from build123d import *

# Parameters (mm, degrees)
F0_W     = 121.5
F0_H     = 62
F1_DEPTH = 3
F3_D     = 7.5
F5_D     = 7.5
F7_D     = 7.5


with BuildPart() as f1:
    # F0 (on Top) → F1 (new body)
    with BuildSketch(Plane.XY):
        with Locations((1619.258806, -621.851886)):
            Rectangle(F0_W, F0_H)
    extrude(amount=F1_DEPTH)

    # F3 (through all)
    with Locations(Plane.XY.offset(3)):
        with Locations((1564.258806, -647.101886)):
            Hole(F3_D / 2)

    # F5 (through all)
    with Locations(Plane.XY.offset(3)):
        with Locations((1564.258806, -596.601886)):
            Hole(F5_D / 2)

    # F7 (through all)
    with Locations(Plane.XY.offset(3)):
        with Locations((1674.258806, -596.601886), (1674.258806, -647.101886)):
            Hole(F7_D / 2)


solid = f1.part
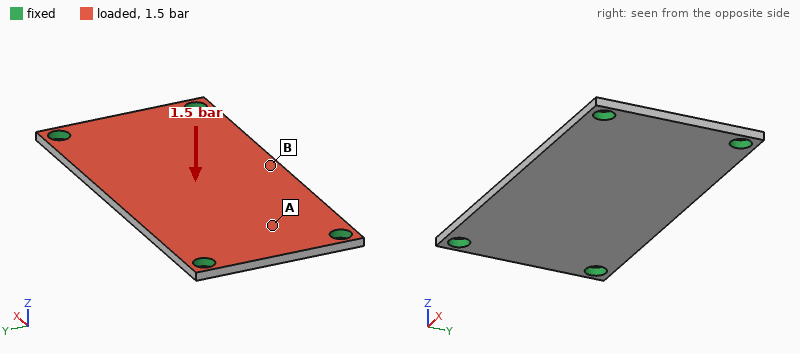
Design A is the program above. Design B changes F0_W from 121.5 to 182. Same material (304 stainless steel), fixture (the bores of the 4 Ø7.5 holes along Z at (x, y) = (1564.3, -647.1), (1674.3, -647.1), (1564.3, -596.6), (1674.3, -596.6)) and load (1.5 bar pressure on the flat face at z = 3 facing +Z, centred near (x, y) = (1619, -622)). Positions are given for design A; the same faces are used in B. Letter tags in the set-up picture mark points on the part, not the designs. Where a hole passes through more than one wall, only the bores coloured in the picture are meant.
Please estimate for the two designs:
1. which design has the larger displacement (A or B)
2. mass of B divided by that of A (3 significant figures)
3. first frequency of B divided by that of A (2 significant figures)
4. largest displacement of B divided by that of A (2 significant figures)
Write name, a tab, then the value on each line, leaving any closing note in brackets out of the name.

which design has the larger displacement	A
mass of B divided by that of A	1.51
first frequency of B divided by that of A	1.0
largest displacement of B divided by that of A	0.91
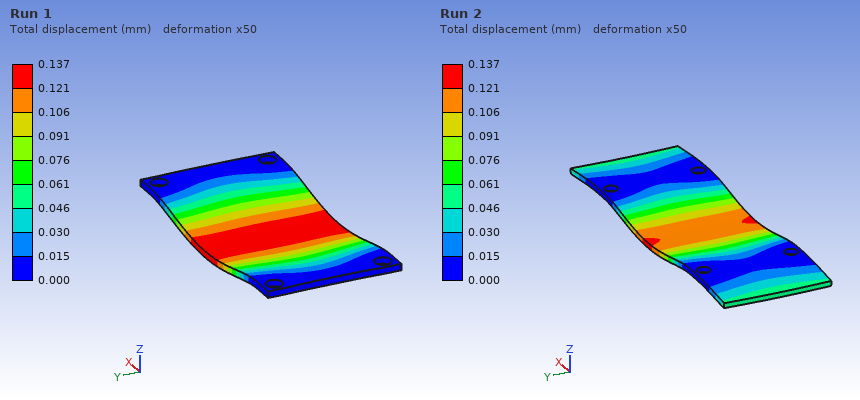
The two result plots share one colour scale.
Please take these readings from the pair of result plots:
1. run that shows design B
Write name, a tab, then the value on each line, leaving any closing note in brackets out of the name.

run that shows design B	Run 2
